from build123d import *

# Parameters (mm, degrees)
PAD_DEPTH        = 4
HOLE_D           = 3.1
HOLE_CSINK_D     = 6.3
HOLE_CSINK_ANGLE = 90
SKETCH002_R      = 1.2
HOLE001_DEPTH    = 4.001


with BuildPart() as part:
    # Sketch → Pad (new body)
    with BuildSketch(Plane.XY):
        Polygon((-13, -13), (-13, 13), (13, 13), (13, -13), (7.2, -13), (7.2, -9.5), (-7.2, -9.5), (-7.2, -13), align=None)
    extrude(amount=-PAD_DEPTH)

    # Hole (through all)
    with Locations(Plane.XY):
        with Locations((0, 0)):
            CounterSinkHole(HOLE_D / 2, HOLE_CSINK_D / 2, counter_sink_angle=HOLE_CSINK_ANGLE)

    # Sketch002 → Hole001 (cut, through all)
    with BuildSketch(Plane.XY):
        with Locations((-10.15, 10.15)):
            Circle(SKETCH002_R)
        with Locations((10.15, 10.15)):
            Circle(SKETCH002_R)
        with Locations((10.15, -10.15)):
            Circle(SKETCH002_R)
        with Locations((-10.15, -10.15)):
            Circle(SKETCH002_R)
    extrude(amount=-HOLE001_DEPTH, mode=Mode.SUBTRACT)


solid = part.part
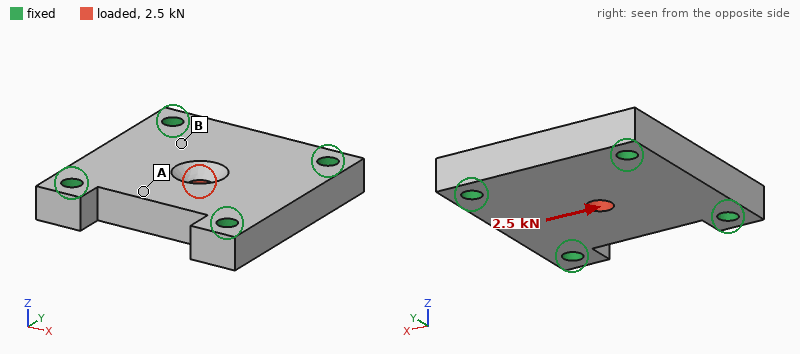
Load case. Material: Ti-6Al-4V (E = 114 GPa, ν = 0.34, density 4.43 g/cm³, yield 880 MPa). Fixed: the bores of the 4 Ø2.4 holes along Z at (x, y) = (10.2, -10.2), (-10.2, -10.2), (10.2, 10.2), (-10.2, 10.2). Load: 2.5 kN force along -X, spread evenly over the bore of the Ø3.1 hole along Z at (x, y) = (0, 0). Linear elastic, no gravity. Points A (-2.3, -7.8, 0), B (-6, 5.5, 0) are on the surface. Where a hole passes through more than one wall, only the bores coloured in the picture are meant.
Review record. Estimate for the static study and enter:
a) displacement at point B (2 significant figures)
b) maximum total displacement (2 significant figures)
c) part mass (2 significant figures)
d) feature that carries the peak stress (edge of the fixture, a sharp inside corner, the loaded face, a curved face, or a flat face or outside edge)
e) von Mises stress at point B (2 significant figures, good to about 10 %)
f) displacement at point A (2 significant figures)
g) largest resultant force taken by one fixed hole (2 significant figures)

1.9 µm
6.3 µm
11 g
the loaded face
27 MPa
1.8 µm
760 N
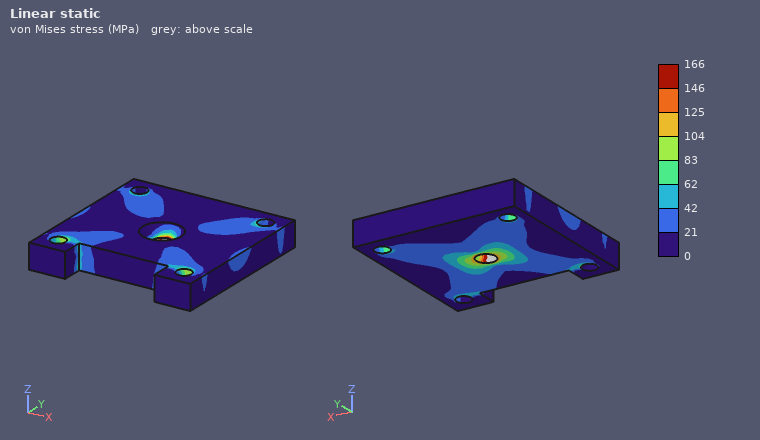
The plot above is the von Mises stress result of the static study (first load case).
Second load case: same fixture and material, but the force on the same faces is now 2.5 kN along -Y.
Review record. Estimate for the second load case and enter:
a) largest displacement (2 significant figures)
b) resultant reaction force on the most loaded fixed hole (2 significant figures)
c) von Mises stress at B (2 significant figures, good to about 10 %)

6.6 µm
760 N
26 MPa
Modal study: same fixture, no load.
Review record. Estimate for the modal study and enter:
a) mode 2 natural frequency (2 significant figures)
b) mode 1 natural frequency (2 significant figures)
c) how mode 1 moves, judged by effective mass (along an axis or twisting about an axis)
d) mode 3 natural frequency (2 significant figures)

46 kHz
29 kHz
along Z
47 kHz
